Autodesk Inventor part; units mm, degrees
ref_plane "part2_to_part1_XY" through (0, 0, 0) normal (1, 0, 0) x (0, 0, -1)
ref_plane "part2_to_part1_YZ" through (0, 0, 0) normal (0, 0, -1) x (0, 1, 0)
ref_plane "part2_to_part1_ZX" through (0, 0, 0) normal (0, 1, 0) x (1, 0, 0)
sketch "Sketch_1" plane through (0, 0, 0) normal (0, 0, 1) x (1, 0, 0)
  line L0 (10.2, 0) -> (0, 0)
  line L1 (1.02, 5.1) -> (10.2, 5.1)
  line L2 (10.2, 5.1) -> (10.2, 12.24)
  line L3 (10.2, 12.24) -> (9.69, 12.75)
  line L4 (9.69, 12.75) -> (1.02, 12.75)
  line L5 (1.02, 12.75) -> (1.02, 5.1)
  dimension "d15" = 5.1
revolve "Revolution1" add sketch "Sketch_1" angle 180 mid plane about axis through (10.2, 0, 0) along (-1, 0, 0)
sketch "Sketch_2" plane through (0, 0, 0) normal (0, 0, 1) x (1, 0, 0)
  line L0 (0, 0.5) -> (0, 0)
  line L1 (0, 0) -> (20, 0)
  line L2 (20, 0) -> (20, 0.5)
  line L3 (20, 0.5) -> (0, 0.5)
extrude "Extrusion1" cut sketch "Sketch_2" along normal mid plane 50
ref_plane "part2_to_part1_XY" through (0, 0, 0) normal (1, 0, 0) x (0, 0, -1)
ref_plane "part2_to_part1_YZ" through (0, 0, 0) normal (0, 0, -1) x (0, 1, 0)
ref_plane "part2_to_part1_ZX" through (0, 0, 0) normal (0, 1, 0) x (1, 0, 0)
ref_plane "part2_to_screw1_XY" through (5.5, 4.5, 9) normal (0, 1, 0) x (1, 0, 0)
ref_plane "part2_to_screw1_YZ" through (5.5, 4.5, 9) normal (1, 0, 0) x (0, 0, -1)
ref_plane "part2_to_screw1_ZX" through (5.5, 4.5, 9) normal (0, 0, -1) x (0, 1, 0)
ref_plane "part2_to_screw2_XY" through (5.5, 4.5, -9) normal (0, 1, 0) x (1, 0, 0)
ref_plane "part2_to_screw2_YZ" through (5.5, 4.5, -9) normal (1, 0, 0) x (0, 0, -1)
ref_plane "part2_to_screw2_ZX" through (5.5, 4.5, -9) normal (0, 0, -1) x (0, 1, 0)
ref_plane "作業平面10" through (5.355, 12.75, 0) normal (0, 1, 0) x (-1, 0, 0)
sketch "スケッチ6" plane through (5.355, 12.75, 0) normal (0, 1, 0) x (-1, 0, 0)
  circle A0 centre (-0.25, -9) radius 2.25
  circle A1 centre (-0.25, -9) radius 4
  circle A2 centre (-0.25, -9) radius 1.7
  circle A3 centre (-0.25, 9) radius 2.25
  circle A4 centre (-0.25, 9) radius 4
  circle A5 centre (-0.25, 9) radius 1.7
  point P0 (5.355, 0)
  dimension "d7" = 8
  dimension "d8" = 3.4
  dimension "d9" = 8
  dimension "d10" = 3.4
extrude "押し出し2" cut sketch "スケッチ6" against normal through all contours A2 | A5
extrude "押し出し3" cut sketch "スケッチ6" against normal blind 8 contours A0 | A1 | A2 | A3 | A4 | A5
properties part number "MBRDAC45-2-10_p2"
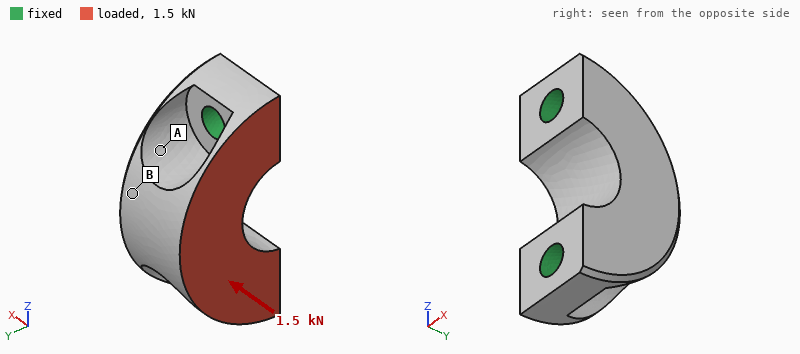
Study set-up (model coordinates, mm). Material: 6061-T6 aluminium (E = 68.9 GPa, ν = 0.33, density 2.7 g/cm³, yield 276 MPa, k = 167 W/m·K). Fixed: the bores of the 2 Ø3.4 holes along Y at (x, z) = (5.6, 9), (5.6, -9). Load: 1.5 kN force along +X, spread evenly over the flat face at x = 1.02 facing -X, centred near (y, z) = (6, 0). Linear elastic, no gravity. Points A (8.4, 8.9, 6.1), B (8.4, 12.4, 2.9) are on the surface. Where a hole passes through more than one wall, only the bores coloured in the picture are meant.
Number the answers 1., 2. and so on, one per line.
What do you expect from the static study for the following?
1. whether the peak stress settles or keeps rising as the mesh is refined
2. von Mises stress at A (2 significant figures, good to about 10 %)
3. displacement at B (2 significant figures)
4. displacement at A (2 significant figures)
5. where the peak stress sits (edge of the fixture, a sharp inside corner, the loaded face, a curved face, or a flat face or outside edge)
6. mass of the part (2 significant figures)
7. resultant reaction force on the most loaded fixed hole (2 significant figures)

1. keeps rising
2. 32 MPa
3. 22 µm
4. 15 µm
5. edge of the fixture
6. 3.9 g
7. 750 N
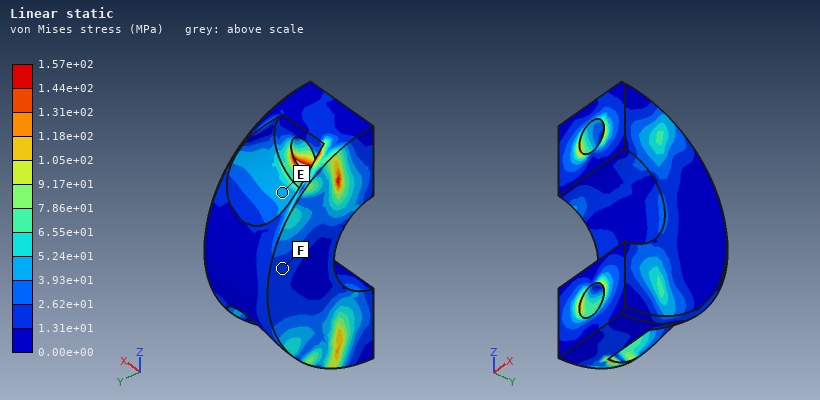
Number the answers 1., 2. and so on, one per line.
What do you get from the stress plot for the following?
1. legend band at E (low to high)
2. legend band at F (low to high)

1. 3.93e+01 to 5.24e+01 MPa
2. 1.31e+01 to 2.62e+01 MPa
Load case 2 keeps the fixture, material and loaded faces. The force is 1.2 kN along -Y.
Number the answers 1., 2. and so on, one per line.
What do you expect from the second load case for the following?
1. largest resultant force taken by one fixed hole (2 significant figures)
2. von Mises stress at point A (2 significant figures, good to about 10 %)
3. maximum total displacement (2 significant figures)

1. 630 N
2. 14 MPa
3. 17 µm
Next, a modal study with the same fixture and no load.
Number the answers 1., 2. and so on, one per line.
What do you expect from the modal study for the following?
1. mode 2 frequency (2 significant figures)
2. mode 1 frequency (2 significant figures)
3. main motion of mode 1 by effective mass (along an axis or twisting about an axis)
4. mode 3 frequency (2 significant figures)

1. 54 kHz
2. 24 kHz
3. along X
4. 54 kHz
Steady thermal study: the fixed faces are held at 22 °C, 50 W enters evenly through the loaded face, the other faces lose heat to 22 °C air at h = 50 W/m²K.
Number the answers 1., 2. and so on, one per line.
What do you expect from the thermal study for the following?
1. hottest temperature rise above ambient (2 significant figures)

1. 27 K
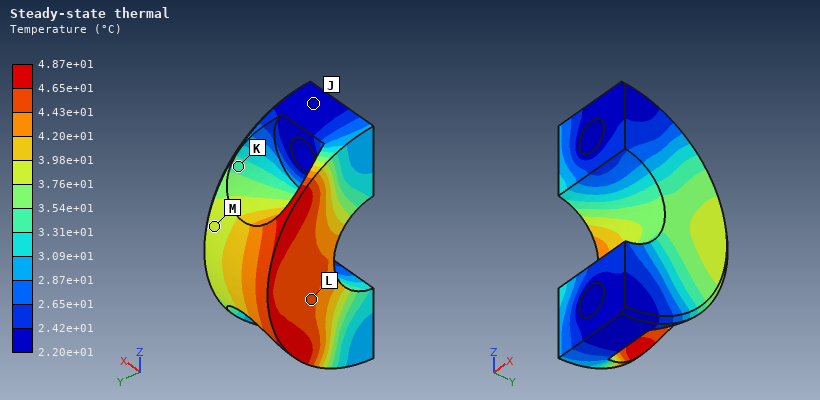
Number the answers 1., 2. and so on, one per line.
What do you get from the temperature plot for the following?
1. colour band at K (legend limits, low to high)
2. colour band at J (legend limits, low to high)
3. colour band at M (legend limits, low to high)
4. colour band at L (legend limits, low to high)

1. 3.31e+01 to 3.54e+01 °C
2. 2.20e+01 to 2.42e+01 °C
3. 3.76e+01 to 3.98e+01 °C
4. 4.43e+01 to 4.65e+01 °C
